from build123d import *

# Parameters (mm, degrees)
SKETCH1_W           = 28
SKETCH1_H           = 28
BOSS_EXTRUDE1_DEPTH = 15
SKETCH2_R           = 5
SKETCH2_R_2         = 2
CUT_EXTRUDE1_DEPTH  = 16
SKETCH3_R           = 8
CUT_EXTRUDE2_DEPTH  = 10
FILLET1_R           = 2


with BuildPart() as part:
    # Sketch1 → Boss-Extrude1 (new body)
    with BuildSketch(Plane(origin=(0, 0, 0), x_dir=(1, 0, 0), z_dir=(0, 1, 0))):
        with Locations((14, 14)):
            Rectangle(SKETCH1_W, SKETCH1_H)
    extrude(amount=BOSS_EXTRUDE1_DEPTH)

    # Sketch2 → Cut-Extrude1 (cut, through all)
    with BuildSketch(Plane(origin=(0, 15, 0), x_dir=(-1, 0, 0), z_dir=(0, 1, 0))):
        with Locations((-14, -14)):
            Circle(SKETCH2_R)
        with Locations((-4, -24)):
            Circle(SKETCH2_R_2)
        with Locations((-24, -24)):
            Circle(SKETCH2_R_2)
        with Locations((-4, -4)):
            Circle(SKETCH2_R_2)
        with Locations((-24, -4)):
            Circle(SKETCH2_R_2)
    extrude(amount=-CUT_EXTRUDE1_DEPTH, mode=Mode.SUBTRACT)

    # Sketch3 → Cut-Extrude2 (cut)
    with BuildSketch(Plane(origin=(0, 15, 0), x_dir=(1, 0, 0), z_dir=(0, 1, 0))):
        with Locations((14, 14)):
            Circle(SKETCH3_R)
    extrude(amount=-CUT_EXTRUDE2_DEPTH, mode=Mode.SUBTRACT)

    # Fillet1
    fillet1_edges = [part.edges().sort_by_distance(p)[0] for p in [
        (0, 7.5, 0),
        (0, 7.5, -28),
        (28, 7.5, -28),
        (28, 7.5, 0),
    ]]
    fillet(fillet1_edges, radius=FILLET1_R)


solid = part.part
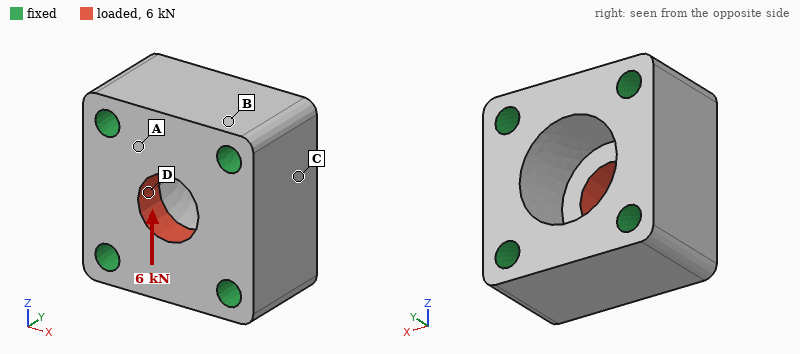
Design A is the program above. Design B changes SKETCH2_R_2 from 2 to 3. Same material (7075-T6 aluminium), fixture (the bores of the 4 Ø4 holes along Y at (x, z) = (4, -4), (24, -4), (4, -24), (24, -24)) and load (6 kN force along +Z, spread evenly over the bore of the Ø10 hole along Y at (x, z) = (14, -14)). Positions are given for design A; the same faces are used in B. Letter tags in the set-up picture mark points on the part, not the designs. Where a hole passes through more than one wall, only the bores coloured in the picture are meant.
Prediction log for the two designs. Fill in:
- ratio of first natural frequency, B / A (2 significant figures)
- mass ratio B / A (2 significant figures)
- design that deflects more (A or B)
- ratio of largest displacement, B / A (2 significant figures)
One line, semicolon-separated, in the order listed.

1.3; 0.89; A; 0.87
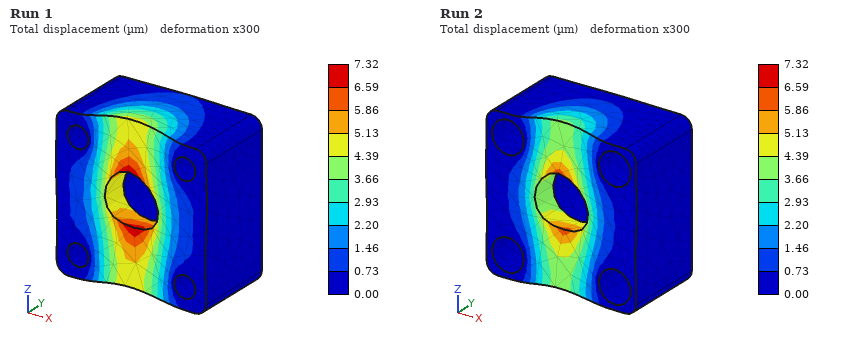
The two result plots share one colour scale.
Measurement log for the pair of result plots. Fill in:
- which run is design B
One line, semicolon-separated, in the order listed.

Run 2
